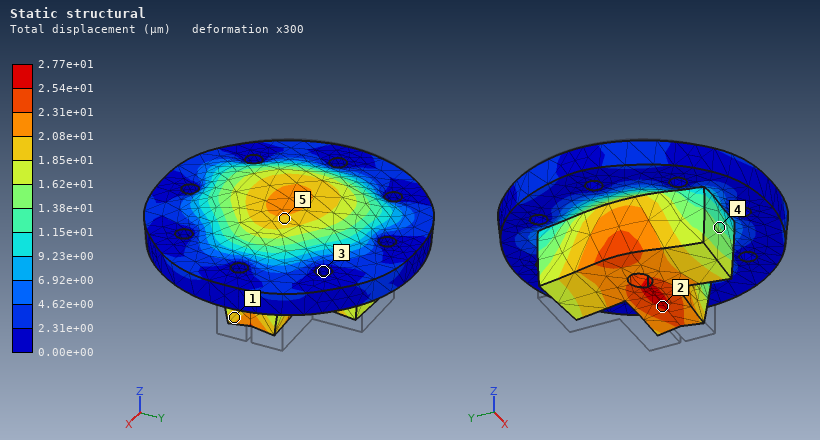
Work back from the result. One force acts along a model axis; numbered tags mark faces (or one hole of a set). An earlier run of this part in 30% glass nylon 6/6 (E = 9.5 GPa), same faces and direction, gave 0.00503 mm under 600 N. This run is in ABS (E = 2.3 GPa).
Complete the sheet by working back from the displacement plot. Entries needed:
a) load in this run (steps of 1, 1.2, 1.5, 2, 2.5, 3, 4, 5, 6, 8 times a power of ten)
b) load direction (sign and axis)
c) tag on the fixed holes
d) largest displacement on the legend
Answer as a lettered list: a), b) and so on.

a) 800 N
b) +Z
c) 3
d) 2.77e+01 µm
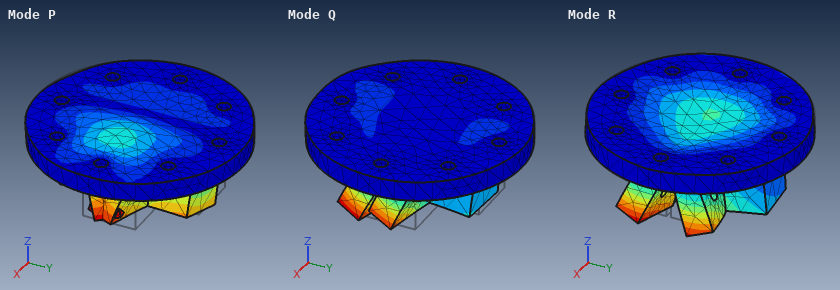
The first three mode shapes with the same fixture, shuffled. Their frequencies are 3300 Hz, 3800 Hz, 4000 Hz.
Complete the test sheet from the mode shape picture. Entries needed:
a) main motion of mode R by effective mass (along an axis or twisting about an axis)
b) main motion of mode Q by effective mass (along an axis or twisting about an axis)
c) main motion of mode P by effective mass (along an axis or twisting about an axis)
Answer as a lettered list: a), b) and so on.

a) along Z
b) along Y
c) along X
